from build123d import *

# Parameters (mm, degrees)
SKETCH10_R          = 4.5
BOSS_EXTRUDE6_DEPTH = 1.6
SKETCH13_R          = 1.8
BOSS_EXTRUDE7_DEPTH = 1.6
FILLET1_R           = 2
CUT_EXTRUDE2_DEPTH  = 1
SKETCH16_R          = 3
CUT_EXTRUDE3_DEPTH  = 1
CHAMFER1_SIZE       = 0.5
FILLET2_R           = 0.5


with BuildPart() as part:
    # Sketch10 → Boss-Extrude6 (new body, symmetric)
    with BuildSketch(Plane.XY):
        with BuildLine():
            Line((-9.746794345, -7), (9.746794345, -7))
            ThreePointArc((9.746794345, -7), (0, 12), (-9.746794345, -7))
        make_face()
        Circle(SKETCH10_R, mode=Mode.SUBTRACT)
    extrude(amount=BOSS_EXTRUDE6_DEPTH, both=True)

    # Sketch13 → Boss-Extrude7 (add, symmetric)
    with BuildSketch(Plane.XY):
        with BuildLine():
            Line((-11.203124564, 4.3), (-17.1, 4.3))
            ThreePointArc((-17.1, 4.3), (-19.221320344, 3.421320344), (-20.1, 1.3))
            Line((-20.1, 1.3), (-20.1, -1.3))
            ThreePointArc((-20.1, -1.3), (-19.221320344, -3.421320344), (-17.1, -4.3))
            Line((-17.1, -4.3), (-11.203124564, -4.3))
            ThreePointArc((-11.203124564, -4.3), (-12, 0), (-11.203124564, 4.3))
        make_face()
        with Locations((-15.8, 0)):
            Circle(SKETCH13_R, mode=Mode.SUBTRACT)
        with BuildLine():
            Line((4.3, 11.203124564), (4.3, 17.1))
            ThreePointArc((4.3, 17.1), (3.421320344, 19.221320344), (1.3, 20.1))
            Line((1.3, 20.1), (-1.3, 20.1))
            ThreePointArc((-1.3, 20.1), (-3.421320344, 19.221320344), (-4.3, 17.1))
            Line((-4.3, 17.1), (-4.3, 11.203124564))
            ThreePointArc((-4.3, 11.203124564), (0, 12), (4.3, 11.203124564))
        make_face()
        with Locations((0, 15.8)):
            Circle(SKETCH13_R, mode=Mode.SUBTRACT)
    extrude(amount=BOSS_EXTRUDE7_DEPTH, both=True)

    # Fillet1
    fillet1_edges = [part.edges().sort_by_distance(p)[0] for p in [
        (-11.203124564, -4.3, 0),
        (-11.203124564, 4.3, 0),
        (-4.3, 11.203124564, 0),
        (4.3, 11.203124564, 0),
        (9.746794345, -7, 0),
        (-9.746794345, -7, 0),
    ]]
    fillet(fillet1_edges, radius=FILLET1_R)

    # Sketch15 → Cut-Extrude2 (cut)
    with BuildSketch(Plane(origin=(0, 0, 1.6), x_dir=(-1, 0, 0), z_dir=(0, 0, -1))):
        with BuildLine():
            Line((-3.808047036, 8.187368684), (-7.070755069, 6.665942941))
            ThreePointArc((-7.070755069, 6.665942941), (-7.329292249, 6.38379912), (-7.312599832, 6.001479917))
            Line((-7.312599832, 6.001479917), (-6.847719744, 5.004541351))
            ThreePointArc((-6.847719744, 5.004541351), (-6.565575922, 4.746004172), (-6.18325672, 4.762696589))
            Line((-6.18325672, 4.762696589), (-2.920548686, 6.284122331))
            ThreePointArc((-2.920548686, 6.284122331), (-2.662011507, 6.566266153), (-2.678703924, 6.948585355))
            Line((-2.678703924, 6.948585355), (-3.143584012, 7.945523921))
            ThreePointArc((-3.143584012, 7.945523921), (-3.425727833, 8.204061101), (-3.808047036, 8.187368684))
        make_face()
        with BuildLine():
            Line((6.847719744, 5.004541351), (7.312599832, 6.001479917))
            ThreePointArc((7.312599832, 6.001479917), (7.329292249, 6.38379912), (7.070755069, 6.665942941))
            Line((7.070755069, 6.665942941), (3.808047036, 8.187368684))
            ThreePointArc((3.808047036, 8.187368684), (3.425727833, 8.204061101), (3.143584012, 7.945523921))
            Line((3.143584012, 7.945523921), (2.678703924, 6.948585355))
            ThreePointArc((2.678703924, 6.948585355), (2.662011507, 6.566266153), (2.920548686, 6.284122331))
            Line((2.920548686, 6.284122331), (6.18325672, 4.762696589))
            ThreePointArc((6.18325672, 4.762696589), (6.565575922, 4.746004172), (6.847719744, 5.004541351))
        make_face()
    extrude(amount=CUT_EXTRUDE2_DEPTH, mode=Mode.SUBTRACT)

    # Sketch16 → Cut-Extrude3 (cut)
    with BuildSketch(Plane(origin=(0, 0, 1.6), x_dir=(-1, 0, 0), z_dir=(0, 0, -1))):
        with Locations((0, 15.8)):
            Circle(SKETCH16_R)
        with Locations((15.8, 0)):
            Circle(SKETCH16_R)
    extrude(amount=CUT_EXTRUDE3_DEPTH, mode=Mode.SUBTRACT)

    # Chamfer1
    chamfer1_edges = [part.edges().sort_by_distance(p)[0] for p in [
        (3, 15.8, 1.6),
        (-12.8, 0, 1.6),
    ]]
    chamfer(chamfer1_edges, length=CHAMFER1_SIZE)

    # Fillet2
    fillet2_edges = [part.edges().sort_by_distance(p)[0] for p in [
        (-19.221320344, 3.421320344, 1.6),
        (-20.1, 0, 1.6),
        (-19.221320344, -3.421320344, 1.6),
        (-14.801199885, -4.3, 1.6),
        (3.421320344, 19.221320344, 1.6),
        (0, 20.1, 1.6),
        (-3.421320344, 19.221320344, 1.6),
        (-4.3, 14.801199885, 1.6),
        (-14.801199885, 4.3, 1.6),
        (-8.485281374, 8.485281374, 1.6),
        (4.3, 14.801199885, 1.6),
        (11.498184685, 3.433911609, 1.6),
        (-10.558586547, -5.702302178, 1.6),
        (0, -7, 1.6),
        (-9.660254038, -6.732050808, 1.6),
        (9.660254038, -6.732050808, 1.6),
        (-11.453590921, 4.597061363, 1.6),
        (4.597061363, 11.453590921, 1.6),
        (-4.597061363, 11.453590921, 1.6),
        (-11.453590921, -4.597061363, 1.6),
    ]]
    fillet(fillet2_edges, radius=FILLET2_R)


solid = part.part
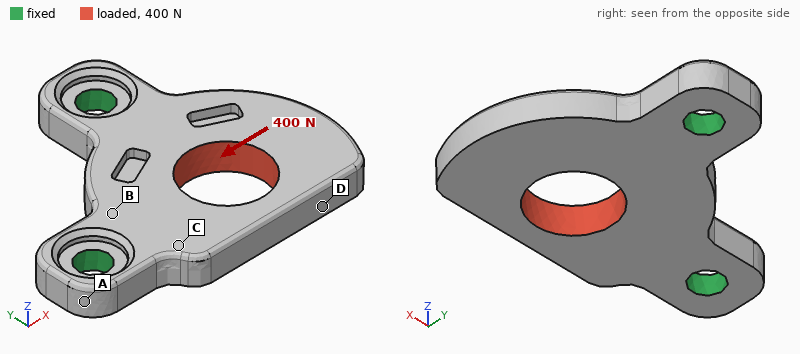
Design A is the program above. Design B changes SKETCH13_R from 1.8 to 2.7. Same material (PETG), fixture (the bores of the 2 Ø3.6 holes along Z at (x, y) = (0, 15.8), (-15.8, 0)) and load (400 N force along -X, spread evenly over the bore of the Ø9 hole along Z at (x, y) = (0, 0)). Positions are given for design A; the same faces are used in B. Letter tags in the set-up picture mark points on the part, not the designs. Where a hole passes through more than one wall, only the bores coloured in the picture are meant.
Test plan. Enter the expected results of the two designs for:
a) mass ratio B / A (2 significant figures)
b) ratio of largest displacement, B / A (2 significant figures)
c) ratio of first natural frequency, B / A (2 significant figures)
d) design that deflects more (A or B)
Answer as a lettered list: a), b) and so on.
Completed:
a) 0.96
b) 0.79
c) 1.2
d) A
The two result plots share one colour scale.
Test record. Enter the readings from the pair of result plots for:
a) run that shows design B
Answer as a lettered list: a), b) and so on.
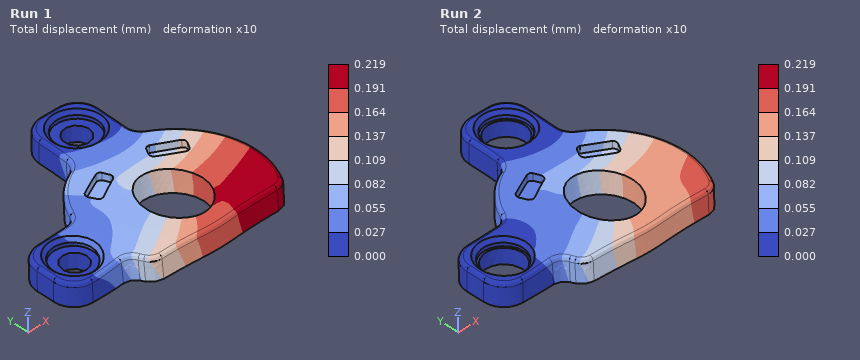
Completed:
a) Run 2
